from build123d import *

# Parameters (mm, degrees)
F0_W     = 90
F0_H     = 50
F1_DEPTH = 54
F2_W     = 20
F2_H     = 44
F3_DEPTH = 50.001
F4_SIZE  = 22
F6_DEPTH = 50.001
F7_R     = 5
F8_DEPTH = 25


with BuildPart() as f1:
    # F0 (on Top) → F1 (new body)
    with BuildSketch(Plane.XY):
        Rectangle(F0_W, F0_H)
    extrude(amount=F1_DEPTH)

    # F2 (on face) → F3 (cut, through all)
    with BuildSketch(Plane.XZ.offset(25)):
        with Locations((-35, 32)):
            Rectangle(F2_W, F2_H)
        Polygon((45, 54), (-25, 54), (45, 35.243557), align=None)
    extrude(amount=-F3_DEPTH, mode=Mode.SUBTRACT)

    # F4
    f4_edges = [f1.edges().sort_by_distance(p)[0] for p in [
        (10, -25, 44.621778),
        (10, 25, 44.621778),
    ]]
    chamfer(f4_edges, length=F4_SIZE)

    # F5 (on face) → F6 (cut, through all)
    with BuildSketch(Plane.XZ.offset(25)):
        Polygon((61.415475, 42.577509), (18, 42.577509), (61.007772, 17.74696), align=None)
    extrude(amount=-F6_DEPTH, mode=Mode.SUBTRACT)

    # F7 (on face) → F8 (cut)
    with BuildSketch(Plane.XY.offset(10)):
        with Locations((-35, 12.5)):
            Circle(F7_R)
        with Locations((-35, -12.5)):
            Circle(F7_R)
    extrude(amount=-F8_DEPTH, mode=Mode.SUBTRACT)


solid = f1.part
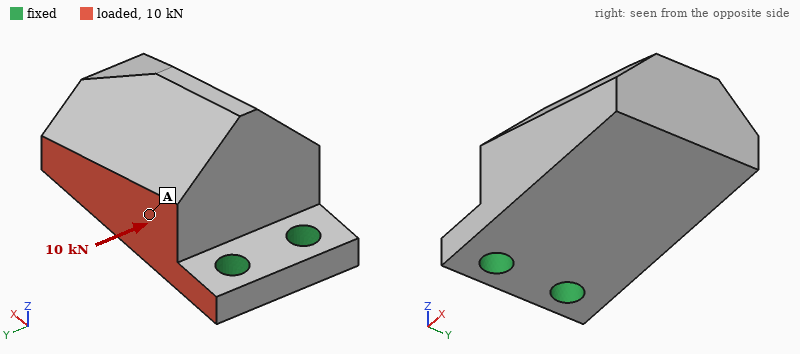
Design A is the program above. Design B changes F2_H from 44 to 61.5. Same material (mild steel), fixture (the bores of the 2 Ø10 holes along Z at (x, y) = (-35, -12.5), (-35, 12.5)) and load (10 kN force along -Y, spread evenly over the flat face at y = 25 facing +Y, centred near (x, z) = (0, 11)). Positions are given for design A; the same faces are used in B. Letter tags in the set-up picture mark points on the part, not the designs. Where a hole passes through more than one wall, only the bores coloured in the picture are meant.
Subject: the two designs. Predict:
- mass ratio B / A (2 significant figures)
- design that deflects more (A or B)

0.94
B
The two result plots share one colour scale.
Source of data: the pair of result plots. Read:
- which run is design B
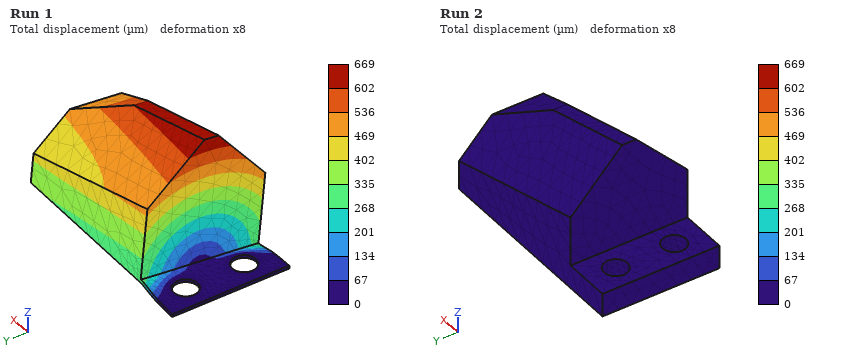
Run 1
